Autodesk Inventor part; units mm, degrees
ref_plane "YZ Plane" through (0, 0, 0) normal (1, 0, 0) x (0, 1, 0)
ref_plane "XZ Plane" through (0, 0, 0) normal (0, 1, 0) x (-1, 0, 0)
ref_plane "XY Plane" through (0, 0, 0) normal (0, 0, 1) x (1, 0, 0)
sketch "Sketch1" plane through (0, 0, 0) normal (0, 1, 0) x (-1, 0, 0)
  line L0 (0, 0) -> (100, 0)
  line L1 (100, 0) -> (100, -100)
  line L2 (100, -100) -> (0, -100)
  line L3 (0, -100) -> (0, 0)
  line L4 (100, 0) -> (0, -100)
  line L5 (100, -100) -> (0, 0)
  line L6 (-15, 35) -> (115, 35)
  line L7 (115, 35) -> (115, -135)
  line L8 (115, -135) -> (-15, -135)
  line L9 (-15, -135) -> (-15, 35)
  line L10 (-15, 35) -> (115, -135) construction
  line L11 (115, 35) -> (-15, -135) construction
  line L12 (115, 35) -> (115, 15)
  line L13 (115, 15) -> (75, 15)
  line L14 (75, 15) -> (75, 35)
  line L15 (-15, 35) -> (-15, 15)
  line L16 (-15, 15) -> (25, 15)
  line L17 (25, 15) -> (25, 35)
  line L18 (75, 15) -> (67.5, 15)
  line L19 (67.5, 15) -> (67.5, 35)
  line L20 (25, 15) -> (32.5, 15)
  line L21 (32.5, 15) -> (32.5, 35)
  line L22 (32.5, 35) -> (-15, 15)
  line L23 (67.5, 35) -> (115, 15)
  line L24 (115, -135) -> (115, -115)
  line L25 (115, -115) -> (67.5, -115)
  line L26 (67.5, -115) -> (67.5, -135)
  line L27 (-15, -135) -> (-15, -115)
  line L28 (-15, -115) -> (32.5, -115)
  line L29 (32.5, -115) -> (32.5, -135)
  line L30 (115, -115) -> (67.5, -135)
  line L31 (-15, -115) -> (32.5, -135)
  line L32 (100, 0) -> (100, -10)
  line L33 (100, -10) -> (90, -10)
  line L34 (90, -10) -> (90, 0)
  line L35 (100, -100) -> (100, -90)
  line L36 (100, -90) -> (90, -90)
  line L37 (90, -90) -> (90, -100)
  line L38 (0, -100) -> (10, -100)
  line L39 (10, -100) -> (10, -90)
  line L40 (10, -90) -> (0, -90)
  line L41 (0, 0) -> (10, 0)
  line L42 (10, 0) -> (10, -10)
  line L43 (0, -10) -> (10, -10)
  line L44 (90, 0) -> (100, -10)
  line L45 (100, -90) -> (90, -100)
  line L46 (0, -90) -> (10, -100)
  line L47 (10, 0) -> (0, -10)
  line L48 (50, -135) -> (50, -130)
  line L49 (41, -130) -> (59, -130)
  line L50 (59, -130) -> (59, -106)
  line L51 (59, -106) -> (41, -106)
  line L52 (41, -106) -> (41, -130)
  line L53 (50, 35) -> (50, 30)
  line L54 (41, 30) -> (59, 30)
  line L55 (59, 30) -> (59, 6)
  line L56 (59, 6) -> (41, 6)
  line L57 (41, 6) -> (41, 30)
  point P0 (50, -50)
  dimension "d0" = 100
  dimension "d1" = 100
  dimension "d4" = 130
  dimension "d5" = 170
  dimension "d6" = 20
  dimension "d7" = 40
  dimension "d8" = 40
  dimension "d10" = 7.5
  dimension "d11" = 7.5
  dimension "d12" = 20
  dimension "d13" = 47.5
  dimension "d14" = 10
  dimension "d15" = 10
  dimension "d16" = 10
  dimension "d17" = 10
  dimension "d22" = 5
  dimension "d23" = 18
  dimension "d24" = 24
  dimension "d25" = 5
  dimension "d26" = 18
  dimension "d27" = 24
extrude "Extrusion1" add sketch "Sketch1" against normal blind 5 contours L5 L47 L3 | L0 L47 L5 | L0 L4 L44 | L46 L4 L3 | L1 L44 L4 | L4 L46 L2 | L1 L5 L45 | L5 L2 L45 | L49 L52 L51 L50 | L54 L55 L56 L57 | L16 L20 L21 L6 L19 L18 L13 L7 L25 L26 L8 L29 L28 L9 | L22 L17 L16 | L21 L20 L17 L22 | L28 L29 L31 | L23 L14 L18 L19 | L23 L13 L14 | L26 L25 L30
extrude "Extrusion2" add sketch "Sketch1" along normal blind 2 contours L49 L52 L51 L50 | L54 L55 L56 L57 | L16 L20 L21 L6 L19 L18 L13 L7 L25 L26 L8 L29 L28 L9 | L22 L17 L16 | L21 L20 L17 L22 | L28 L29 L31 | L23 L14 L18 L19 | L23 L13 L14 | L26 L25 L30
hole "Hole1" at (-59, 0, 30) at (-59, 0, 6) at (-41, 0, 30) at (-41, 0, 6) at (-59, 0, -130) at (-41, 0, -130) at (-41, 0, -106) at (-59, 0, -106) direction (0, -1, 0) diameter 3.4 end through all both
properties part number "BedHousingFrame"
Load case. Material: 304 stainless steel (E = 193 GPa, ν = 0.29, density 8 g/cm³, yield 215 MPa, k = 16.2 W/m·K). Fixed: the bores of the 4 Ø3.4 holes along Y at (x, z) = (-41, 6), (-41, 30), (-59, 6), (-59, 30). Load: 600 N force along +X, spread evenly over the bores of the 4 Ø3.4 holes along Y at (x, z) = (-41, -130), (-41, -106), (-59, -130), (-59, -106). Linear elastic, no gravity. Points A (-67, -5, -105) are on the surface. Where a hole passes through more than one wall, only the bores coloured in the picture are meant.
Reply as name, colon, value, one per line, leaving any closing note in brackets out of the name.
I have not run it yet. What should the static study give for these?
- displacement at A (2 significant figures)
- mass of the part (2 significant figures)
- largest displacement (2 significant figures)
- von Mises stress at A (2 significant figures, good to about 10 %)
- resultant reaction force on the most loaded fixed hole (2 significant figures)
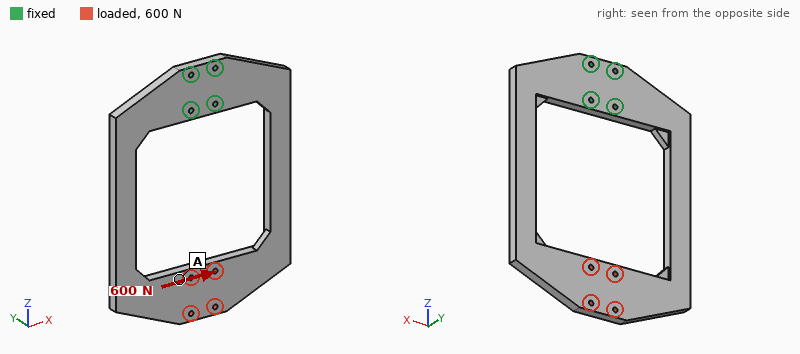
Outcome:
displacement at A: 0.13 mm
mass of the part: 580 g
largest displacement: 0.13 mm
von Mises stress at A: 5.5 MPa
resultant reaction force on the most loaded fixed hole: 1.6 kN
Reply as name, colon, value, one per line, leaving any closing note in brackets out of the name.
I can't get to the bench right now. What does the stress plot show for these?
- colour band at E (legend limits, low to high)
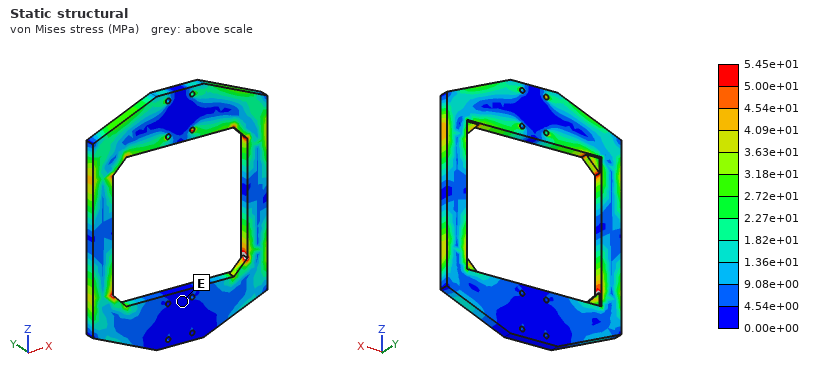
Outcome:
colour band at E: 0.00e+00 to 4.54e+00 MPa
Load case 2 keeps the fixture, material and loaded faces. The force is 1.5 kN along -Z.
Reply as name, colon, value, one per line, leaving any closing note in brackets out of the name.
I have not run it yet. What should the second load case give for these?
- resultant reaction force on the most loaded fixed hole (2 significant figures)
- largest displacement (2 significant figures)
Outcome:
resultant reaction force on the most loaded fixed hole: 1.2 kN
largest displacement: 28 µm
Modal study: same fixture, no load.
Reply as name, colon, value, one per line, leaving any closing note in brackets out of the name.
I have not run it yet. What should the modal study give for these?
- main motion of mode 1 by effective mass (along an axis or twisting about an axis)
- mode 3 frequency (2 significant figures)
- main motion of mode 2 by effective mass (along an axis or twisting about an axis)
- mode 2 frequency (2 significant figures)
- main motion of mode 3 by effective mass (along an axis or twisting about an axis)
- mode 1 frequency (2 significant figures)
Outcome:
main motion of mode 1 by effective mass: along Y
mode 3 frequency: 670 Hz
main motion of mode 2 by effective mass: twisting about Z
mode 2 frequency: 400 Hz
main motion of mode 3 by effective mass: along X
mode 1 frequency: 150 Hz
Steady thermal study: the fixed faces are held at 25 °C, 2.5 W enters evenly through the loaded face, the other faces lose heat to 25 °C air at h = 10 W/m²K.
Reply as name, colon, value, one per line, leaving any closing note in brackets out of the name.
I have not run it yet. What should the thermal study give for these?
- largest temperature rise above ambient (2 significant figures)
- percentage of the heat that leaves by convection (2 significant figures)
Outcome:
largest temperature rise above ambient: 25 K
percentage of the heat that leaves by convection: 93 %
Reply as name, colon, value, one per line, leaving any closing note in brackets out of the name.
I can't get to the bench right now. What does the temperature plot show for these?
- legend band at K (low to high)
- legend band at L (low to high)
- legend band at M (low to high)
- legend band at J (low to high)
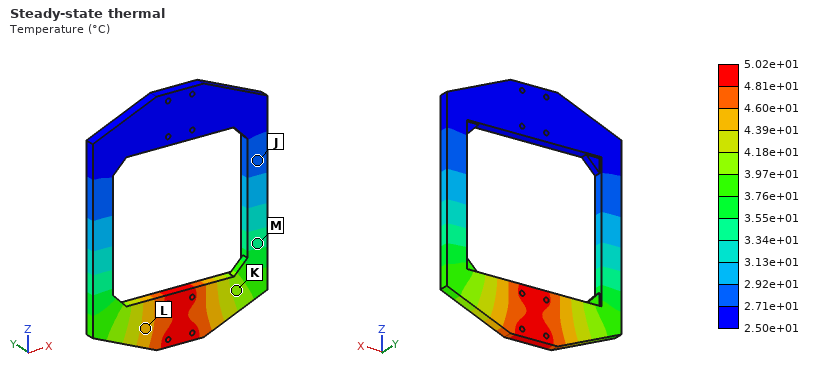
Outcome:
legend band at K: 3.97e+01 to 4.18e+01 °C
legend band at L: 4.39e+01 to 4.60e+01 °C
legend band at M: 3.34e+01 to 3.55e+01 °C
legend band at J: 2.71e+01 to 2.92e+01 °C
